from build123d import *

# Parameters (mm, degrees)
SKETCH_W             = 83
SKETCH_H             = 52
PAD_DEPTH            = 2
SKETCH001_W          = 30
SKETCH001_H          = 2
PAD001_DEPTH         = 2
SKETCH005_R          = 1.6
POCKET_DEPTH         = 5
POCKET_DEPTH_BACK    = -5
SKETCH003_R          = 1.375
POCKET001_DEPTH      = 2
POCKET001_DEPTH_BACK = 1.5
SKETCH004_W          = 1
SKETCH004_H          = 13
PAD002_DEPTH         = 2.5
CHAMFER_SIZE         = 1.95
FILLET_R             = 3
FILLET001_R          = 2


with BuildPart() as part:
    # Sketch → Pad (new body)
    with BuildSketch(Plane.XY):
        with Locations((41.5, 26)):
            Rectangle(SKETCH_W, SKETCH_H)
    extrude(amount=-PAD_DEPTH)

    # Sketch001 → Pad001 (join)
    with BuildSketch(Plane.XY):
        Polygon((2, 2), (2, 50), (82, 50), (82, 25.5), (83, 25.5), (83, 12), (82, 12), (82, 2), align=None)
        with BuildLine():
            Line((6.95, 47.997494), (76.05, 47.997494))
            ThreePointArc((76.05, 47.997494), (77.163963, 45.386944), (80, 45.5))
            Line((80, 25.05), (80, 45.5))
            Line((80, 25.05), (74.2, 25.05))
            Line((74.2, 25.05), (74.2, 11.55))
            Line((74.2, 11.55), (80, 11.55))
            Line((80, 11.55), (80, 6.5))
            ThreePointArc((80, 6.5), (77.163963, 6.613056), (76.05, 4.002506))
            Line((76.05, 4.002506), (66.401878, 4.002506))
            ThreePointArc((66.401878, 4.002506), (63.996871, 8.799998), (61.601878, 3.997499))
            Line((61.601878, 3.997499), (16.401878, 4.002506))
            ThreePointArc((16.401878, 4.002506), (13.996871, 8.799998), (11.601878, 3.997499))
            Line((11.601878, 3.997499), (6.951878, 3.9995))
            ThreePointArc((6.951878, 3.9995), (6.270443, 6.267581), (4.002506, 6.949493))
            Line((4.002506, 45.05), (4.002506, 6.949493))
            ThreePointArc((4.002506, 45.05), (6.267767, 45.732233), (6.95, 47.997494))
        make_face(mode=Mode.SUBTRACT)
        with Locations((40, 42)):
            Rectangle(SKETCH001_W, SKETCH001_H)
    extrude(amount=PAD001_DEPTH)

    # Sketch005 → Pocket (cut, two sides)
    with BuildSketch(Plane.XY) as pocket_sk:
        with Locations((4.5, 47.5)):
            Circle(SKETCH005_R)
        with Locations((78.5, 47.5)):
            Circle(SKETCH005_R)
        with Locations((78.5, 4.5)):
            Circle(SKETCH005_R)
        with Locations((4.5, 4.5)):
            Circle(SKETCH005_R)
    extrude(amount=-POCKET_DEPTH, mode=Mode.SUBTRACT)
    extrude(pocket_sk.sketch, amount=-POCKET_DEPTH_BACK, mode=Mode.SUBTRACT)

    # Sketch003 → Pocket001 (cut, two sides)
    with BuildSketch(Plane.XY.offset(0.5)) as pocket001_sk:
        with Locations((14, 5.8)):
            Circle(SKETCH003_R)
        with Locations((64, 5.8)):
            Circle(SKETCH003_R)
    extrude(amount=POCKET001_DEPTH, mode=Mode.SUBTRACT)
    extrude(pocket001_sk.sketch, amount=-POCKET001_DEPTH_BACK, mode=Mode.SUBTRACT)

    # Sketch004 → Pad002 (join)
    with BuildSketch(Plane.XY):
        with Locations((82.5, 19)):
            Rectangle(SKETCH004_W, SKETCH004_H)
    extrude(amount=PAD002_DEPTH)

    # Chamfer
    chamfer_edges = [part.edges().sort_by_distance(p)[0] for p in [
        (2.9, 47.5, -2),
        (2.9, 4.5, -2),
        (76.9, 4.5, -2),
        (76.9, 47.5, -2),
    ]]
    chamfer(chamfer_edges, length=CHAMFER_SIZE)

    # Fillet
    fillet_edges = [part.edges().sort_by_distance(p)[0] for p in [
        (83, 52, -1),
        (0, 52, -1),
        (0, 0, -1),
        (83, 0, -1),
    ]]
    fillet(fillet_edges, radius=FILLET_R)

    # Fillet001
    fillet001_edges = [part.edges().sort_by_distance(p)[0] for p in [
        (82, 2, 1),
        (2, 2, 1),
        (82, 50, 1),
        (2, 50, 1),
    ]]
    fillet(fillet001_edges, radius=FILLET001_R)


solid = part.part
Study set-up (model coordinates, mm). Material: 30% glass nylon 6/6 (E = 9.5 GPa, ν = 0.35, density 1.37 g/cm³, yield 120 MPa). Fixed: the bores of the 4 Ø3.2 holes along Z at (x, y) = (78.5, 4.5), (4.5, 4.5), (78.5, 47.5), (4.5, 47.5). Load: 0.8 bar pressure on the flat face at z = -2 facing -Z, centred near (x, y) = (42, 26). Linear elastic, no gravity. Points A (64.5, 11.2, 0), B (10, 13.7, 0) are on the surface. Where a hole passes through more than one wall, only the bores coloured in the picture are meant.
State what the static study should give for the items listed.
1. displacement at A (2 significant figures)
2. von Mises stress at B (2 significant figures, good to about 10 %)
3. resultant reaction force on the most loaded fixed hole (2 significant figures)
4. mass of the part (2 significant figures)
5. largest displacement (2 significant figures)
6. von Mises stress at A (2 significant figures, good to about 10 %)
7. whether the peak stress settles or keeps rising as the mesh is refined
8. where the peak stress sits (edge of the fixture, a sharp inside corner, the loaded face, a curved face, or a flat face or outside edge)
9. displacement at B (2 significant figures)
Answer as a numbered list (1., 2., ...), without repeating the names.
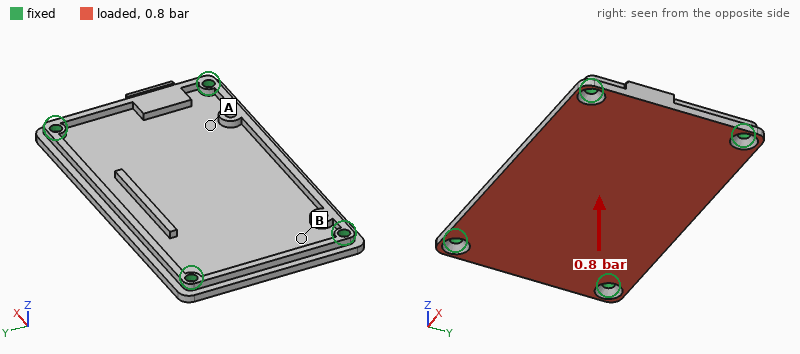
1. 0.36 mm
2. 11 MPa
3. 210 N
4. 13 g
5. 0.81 mm
6. 5.0 MPa
7. keeps rising
8. edge of the fixture
9. 0.17 mm
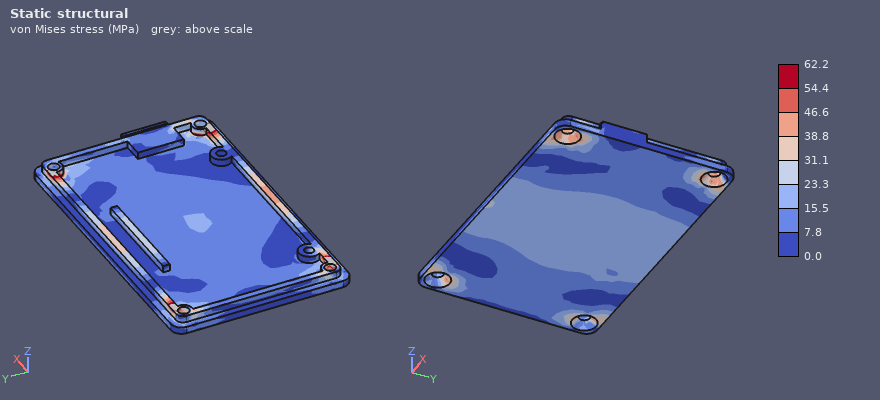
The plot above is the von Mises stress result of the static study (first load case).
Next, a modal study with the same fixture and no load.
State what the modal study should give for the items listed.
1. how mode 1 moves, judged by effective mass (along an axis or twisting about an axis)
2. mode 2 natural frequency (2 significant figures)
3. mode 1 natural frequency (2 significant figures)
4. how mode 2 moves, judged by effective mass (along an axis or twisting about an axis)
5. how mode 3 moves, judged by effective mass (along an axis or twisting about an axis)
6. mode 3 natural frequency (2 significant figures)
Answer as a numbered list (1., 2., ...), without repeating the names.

1. along Z
2. 1700 Hz
3. 1100 Hz
4. twisting about X
5. twisting about Y
6. 2600 Hz
